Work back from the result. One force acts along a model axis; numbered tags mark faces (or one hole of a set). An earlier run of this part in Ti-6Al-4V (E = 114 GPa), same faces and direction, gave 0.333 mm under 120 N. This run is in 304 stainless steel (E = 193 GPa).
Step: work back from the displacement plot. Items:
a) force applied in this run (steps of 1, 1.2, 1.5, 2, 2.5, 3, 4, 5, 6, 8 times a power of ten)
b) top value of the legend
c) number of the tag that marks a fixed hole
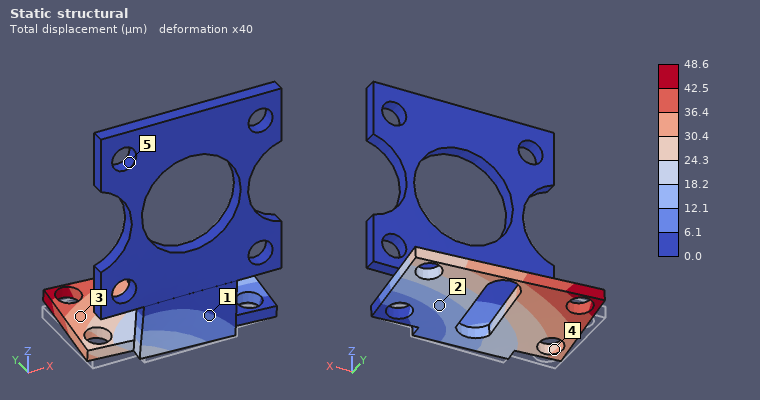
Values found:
30 N
48.6 µm
5
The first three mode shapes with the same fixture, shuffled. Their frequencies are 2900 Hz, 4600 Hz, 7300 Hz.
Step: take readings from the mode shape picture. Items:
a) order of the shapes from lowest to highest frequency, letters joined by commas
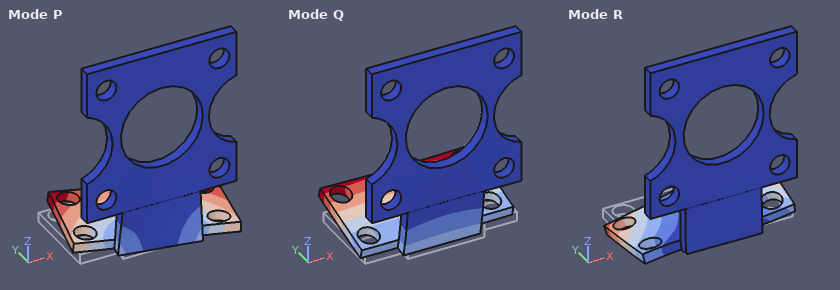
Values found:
Q, P, R
